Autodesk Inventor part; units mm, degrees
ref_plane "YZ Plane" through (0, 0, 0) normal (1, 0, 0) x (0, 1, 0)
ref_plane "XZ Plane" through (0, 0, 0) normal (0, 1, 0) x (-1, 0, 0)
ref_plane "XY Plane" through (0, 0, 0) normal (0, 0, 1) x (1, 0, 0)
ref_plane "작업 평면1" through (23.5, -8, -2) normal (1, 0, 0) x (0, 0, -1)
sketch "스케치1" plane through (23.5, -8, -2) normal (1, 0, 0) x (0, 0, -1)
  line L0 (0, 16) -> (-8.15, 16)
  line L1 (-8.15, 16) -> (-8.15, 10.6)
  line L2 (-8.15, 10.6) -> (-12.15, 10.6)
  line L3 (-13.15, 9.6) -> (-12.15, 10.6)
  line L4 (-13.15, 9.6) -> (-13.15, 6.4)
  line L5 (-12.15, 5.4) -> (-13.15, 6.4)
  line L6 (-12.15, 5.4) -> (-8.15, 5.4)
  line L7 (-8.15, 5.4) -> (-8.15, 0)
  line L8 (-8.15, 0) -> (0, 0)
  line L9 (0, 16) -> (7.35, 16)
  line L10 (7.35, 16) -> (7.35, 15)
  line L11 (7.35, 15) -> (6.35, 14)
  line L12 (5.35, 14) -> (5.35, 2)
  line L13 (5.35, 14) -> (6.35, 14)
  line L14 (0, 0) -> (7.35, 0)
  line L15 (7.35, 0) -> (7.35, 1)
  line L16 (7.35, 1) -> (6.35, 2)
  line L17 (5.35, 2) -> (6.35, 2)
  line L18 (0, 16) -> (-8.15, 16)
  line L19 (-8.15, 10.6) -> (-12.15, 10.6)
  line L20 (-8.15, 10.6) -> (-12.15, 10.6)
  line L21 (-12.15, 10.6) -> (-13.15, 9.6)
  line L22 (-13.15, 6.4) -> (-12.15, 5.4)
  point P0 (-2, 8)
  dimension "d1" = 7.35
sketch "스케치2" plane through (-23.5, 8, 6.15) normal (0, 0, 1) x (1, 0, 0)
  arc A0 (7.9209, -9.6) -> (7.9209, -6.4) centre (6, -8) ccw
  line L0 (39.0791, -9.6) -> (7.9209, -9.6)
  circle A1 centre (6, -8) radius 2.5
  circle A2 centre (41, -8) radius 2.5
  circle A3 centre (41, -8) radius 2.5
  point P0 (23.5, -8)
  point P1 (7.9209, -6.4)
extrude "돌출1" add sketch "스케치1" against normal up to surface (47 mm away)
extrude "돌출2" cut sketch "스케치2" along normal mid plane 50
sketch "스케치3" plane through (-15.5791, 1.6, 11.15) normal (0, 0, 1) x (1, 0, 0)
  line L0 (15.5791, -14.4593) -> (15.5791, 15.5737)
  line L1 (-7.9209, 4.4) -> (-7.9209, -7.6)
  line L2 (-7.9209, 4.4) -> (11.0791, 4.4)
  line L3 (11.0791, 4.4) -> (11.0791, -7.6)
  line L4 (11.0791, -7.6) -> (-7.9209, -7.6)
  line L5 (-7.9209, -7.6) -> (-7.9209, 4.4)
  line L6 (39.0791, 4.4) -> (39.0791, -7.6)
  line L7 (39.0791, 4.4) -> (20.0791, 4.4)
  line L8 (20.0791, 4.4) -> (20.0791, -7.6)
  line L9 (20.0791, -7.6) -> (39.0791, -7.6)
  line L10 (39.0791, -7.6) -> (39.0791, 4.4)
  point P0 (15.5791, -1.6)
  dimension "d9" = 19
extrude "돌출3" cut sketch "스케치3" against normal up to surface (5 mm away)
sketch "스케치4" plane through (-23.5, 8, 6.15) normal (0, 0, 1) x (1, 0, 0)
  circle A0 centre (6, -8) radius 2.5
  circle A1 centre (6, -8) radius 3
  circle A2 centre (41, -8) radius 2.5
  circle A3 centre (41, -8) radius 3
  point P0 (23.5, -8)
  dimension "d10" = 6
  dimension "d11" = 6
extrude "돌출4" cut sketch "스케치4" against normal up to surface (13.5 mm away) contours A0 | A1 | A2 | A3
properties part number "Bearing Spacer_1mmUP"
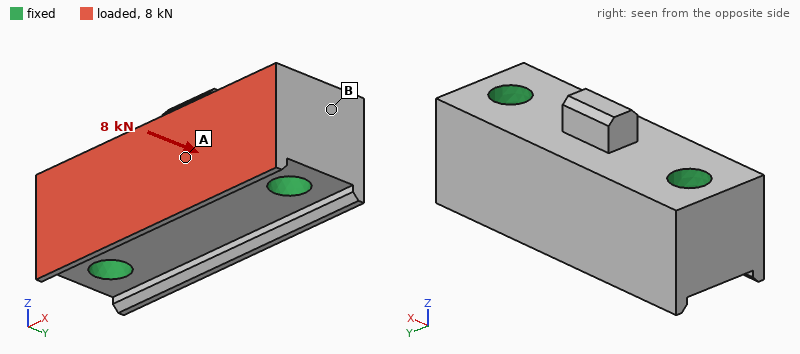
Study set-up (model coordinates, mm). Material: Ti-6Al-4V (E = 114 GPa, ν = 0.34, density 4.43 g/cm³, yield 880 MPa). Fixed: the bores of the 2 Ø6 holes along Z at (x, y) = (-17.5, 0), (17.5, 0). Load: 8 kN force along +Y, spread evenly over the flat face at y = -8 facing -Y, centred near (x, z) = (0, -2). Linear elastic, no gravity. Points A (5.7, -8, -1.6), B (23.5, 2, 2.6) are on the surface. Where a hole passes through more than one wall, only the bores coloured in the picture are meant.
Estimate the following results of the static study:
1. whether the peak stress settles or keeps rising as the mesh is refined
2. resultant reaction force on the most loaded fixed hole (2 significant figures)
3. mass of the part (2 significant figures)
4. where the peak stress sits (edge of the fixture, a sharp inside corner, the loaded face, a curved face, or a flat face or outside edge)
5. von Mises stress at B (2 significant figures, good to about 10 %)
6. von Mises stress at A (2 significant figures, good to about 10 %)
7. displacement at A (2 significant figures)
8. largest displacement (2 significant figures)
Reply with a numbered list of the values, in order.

1. keeps rising
2. 4.0 kN
3. 44 g
4. edge of the fixture
5. 6.6 MPa
6. 21 MPa
7. 4.2 µm
8. 8.3 µm
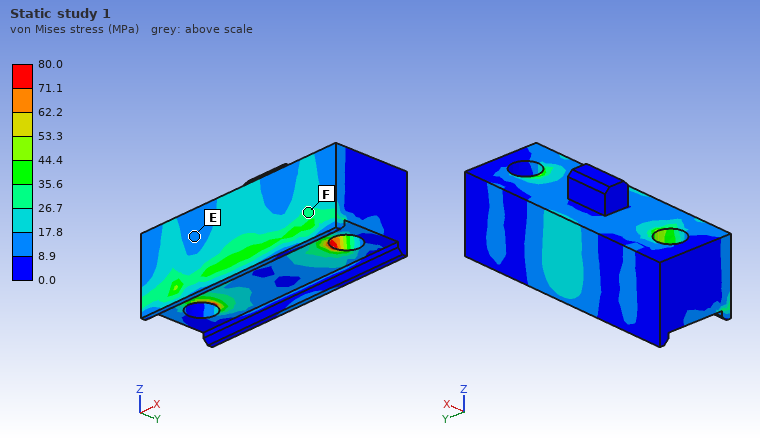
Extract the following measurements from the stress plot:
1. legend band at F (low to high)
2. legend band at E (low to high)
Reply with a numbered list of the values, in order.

1. 26.7 to 35.6 MPa
2. 8.9 to 17.8 MPa
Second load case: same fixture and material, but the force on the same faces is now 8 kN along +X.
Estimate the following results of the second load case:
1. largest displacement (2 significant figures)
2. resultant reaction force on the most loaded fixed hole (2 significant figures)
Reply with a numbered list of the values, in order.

1. 5.4 µm
2. 4.2 kN
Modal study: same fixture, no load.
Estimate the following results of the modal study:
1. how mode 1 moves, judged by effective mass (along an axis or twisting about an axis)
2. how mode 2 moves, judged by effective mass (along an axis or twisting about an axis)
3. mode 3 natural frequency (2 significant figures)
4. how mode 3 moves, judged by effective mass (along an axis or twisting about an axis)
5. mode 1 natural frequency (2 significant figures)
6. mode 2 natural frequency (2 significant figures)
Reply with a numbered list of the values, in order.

1. along Y
2. along Z
3. 38 kHz
4. twisting about X
5. 33 kHz
6. 35 kHz
